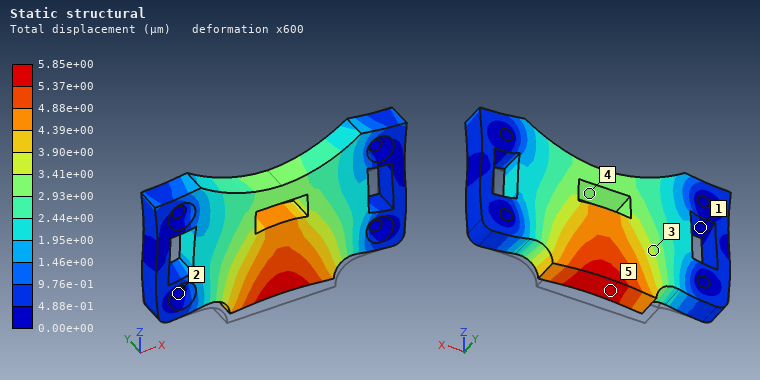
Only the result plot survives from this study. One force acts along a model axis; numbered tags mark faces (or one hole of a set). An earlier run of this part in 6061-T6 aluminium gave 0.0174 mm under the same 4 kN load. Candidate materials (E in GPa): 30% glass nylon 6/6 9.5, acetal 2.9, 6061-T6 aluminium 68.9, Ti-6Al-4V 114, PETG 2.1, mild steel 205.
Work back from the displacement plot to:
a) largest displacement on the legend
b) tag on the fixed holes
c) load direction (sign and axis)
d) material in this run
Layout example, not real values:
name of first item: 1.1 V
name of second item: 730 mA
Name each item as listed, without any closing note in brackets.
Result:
largest displacement on the legend: 5.85e+00 µm
tag on the fixed holes: 2
load direction: +Z
material in this run: mild steel
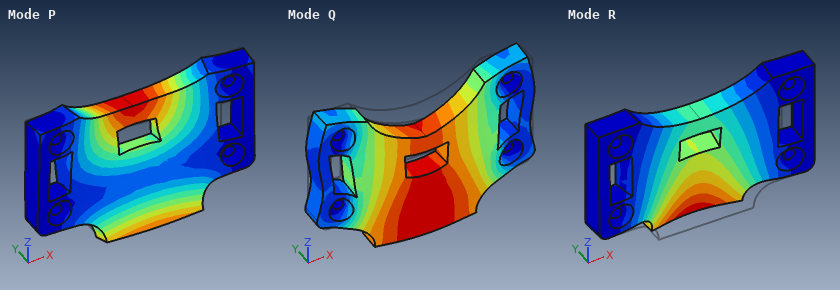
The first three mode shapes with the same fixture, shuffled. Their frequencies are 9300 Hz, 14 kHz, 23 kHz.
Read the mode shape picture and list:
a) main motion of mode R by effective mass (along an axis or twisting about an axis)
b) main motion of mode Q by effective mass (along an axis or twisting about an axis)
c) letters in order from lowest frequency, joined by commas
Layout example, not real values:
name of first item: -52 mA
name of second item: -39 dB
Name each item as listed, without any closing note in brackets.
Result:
main motion of mode R by effective mass: along Y
main motion of mode Q by effective mass: along Z
letters in order from lowest frequency, joined by commas: R, P, Q
